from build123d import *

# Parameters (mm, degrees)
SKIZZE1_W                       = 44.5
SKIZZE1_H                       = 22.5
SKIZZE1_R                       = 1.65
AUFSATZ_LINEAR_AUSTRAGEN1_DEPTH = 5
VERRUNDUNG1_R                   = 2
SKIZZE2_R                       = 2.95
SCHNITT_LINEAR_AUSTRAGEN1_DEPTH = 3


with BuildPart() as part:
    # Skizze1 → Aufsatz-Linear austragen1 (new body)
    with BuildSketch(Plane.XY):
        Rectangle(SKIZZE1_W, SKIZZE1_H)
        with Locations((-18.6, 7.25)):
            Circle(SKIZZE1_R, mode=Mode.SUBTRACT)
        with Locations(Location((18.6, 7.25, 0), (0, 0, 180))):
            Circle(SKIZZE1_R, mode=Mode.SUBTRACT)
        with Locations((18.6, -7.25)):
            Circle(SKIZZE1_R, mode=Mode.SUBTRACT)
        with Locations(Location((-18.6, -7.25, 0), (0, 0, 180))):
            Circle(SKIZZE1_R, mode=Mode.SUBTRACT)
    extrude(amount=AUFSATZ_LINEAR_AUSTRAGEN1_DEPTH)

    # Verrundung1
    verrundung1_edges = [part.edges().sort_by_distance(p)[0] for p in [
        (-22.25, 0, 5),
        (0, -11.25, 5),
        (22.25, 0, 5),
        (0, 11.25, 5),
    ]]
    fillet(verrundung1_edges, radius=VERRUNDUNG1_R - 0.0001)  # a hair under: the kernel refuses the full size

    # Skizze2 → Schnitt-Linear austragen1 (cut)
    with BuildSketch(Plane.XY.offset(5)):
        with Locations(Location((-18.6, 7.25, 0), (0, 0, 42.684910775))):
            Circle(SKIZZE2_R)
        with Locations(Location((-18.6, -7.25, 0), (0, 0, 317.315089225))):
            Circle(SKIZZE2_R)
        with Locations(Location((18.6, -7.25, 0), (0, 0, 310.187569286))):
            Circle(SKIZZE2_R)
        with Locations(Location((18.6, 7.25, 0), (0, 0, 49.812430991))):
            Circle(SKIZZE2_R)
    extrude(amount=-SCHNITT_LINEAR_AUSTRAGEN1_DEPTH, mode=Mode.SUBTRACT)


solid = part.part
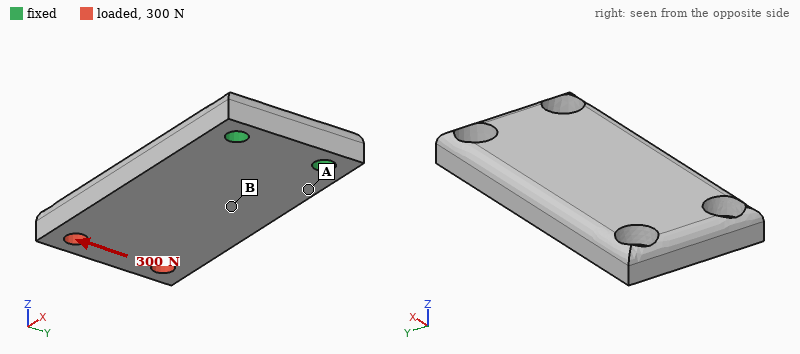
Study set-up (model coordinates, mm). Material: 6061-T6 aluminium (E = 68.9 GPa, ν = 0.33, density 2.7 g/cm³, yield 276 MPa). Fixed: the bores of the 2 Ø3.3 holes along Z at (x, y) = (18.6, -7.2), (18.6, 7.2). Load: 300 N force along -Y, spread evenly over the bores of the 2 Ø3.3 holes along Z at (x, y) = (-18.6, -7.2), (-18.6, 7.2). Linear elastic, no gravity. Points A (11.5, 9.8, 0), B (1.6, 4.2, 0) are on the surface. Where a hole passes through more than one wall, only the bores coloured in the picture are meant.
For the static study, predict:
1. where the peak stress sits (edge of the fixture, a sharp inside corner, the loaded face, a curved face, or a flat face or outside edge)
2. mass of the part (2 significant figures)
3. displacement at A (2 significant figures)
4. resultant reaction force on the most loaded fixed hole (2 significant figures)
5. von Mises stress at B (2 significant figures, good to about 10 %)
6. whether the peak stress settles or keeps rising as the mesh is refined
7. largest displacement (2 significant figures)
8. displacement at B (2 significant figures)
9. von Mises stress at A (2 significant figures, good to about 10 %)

edge of the fixture
12 g
7.1 µm
700 N
14 MPa
keeps rising
41 µm
13 µm
28 MPa
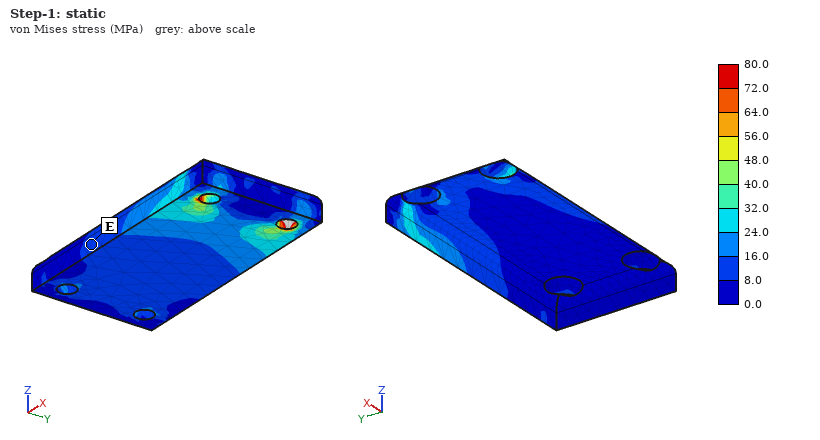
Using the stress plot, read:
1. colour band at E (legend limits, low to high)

8.0 to 16.0 MPa
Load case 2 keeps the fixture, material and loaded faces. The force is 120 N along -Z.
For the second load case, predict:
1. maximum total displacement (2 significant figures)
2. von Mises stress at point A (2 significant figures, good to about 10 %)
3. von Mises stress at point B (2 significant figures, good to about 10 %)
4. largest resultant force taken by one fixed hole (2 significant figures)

0.28 mm
37 MPa
27 MPa
64 N
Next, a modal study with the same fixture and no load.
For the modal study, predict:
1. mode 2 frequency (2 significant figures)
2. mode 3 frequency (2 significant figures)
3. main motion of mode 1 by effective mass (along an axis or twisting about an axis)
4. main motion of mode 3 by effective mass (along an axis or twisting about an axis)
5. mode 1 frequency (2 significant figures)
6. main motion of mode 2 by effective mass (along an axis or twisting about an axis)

7600 Hz
9300 Hz
along Z
along Y
1800 Hz
along Y
